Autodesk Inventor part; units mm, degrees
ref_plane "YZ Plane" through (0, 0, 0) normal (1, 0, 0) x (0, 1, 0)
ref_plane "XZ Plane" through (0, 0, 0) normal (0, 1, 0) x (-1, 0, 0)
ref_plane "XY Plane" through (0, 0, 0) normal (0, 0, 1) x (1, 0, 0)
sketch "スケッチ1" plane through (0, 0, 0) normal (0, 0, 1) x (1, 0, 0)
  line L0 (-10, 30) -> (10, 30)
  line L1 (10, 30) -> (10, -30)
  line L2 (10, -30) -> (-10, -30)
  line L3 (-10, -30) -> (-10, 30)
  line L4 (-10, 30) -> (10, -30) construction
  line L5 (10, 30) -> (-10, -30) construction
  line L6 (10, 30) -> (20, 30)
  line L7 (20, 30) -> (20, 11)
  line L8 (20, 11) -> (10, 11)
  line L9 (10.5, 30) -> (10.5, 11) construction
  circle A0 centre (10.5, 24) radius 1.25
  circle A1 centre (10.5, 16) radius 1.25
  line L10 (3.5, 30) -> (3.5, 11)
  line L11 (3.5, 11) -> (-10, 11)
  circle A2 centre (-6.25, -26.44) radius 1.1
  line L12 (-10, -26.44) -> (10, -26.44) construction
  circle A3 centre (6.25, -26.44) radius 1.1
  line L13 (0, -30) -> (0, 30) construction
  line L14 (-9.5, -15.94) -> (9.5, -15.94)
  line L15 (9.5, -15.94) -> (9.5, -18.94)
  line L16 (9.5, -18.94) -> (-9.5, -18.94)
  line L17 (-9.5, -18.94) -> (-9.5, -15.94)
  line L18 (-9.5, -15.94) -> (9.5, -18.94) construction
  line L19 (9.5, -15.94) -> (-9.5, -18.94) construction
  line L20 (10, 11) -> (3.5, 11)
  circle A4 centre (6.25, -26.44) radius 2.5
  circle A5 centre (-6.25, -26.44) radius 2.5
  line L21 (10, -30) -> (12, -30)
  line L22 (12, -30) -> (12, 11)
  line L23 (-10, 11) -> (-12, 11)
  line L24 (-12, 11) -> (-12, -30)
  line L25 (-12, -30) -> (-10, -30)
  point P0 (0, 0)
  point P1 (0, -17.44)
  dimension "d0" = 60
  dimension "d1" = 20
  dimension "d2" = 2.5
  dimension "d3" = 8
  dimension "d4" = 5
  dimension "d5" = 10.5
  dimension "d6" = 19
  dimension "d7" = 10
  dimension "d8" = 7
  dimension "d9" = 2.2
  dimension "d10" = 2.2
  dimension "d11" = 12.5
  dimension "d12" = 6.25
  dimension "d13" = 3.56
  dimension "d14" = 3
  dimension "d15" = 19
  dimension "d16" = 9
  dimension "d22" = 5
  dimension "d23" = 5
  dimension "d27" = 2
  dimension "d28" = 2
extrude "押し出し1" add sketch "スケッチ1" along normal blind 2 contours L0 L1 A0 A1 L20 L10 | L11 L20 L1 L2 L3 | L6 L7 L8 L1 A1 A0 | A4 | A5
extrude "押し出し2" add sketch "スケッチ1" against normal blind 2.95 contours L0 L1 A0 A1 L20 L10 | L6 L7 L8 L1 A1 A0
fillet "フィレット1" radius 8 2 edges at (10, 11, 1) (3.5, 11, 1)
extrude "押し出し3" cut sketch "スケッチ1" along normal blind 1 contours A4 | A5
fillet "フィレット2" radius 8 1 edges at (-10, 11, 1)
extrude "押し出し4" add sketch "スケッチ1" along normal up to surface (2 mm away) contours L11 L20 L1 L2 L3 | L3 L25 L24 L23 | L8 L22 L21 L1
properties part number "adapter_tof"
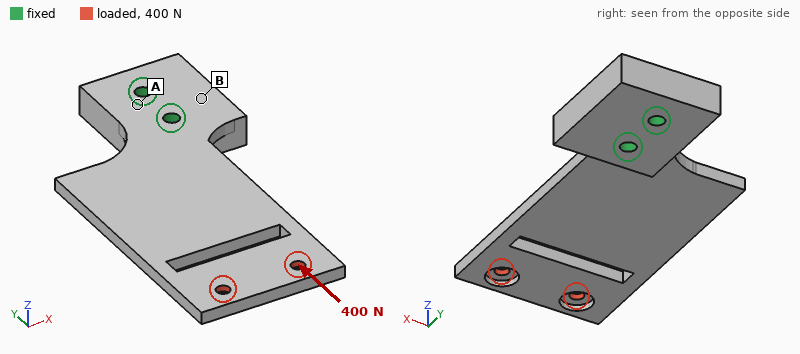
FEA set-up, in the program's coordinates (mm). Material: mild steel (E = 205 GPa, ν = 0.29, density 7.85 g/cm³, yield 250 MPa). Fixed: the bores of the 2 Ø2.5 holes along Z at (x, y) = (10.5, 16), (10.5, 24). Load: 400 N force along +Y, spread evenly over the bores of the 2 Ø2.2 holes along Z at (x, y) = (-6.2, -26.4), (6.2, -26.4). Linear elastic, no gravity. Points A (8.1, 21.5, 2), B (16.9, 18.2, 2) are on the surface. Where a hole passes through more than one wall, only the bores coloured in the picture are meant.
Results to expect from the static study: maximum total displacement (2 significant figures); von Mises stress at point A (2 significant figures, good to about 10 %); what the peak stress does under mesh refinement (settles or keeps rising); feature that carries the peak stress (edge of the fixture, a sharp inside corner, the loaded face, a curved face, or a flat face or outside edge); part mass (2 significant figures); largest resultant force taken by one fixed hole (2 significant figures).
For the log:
0.11 mm
21 MPa
keeps rising
a sharp inside corner
26 g
430 N
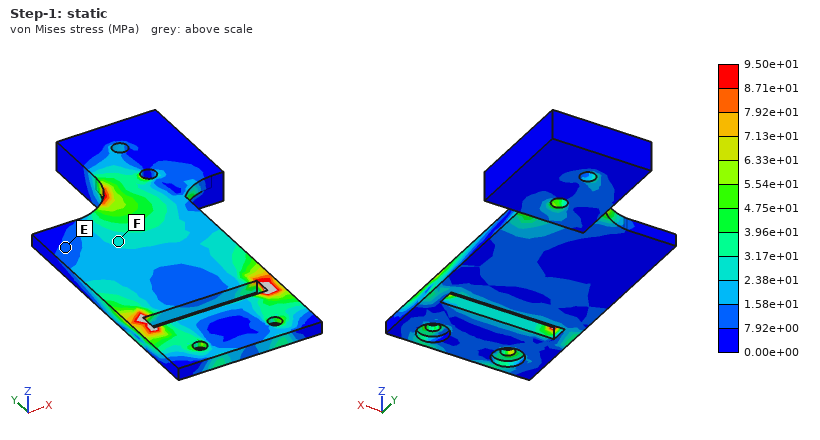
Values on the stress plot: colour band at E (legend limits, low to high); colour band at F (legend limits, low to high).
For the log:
7.92e+00 to 1.58e+01 MPa
2.38e+01 to 3.17e+01 MPa
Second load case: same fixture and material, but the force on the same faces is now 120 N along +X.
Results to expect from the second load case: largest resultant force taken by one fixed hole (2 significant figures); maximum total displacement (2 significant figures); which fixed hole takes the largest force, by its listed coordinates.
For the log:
590 N
48 µm
(10.5, 16)
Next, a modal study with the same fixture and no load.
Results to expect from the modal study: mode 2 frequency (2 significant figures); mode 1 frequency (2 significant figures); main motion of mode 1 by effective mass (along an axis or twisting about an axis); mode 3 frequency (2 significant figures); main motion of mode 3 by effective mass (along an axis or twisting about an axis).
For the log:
2600 Hz
790 Hz
along Z
3600 Hz
along X
